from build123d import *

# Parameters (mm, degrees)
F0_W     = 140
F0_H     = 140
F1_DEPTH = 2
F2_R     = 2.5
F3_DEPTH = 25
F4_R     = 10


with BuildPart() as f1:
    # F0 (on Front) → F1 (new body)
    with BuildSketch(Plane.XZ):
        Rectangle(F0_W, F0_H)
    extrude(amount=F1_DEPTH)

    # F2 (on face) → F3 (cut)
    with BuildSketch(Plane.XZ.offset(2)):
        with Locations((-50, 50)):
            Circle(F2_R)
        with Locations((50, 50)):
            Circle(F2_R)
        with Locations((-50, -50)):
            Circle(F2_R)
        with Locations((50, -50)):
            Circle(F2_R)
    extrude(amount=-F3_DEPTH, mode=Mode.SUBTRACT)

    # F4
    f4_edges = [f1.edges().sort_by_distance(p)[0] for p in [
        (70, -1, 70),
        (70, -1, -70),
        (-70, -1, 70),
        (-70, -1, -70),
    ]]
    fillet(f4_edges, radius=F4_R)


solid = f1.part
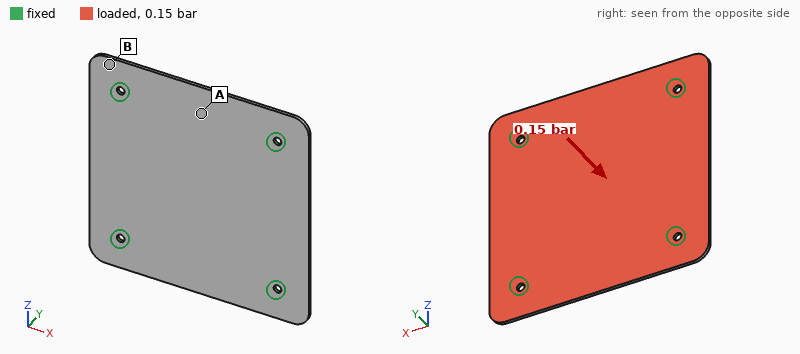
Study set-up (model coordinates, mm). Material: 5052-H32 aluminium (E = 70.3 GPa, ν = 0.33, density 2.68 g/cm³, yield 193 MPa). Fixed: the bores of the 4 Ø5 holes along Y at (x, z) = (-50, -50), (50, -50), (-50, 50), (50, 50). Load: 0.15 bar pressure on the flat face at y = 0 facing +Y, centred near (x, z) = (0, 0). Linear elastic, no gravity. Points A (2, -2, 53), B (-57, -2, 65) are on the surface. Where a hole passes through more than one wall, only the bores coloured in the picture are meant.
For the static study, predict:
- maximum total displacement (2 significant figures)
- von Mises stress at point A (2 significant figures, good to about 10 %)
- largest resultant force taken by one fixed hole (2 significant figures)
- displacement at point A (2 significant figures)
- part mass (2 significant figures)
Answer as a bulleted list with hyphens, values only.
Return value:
- 0.19 mm
- 11 MPa
- 73 N
- 0.11 mm
- 100 g
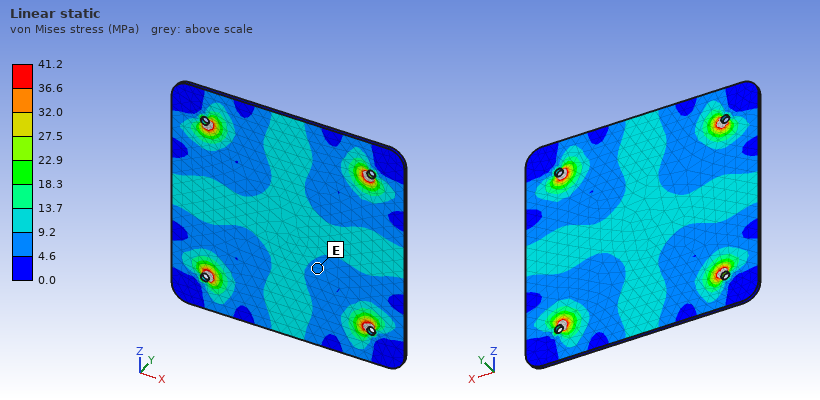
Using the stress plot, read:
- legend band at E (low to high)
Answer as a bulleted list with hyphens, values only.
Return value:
- 4.6 to 9.2 MPa
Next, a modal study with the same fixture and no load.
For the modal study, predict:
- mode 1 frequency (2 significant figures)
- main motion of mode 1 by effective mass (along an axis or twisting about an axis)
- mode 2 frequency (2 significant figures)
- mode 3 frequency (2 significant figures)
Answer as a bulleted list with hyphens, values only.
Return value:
- 740 Hz
- along Y
- 1100 Hz
- 1100 Hz
